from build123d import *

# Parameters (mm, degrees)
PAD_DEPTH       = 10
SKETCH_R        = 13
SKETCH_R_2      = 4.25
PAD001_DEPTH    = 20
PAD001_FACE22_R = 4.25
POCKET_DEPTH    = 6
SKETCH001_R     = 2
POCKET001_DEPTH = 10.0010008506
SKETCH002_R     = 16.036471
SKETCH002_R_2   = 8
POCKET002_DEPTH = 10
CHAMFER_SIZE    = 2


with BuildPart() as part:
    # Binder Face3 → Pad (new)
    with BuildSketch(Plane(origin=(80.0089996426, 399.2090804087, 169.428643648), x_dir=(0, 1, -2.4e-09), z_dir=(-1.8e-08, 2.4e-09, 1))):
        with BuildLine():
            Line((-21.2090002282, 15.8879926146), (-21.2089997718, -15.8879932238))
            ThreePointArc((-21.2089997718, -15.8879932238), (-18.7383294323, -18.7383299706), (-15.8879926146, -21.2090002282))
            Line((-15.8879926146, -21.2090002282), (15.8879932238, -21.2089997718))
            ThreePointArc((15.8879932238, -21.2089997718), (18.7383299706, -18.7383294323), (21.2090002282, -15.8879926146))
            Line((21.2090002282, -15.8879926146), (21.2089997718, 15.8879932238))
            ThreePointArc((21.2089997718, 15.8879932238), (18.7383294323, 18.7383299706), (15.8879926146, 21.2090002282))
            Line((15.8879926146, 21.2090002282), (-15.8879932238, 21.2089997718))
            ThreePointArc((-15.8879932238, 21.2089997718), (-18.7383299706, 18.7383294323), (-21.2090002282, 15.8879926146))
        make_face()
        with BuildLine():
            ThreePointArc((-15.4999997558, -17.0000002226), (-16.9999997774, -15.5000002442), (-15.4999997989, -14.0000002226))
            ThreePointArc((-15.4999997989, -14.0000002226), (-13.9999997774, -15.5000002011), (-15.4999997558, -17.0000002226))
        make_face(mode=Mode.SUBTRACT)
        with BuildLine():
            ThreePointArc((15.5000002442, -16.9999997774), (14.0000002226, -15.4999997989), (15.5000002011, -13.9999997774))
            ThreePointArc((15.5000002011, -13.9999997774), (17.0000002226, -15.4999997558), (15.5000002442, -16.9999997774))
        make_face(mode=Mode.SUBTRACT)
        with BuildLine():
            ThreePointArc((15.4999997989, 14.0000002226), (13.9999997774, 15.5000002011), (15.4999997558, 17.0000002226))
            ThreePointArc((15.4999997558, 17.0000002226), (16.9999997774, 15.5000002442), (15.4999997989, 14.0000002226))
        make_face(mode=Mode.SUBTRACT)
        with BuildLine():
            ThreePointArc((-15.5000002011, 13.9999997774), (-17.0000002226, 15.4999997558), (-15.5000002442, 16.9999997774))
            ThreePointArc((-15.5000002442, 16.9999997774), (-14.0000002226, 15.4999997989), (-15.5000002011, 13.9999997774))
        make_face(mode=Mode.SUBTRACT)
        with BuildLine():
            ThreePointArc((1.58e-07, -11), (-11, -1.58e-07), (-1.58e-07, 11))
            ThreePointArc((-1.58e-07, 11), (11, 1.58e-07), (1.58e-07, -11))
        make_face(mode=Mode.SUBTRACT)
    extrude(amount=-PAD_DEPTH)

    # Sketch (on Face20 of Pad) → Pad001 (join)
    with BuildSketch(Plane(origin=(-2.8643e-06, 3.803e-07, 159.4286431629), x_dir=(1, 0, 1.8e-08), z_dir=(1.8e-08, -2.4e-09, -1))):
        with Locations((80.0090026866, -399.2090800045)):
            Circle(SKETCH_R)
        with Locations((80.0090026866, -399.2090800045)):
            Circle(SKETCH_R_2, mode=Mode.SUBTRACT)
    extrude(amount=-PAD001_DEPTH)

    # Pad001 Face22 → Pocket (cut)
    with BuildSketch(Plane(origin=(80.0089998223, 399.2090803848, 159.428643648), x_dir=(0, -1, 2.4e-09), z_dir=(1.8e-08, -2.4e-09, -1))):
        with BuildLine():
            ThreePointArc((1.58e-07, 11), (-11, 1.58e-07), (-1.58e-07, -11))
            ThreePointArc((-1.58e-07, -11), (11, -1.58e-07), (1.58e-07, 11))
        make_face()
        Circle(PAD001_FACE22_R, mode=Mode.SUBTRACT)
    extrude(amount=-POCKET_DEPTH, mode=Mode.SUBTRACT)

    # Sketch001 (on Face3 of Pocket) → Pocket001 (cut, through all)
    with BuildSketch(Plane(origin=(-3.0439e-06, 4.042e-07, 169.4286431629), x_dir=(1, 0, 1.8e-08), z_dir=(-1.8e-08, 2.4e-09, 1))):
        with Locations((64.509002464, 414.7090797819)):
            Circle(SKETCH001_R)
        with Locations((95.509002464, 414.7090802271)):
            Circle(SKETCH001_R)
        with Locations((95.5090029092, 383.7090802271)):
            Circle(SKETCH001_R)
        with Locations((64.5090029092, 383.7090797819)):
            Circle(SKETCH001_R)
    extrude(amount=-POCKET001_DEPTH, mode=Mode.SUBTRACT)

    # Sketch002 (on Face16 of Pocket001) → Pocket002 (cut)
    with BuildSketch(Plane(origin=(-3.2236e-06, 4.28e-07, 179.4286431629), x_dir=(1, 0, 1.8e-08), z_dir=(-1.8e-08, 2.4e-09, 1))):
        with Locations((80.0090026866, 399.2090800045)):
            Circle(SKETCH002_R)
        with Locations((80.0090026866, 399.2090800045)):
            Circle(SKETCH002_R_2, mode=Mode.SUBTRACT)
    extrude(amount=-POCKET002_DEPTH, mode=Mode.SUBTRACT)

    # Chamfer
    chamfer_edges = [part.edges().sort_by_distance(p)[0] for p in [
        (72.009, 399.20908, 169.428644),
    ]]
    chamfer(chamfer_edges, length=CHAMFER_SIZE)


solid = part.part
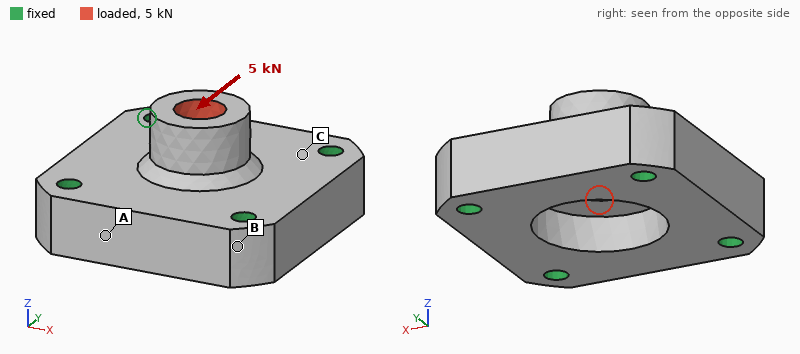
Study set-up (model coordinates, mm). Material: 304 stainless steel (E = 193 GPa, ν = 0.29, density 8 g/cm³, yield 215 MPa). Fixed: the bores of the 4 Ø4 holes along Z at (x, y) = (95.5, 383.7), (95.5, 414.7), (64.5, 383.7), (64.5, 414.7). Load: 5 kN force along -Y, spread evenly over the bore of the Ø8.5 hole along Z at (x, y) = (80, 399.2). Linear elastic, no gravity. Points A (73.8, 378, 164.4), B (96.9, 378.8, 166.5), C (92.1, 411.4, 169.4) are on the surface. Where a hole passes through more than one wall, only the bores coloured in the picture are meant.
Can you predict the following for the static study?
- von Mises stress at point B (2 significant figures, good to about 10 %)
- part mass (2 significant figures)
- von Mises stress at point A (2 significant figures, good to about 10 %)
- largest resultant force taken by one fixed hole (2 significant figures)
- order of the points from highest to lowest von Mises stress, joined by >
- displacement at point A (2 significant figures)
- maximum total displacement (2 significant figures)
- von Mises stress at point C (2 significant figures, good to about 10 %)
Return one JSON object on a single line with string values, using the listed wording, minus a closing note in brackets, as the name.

{"von Mises stress at point B": "5.9 MPa", "part mass": "130 g", "von Mises stress at point A": "10.0 MPa", "largest resultant force taken by one fixed hole": "1.5 kN", "order of the points from highest to lowest von Mises stress, joined by >": "C > A > B", "displacement at point A": "1.2 µm", "maximum total displacement": "7.6 µm", "von Mises stress at point C": "20 MPa"}
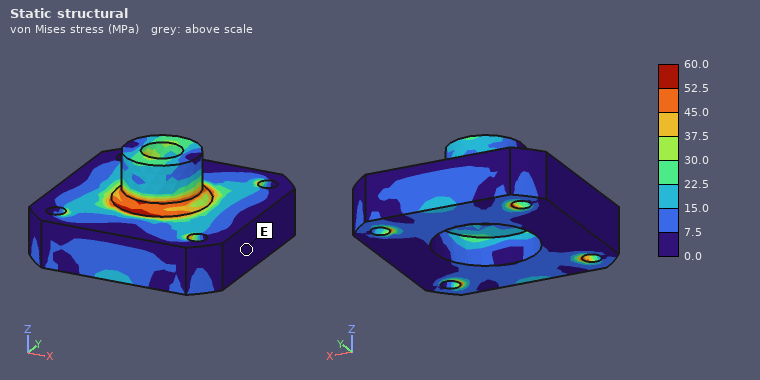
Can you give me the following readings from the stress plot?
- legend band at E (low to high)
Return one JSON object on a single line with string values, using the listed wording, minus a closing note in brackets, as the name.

{"legend band at E": "0.0 to 7.5 MPa"}
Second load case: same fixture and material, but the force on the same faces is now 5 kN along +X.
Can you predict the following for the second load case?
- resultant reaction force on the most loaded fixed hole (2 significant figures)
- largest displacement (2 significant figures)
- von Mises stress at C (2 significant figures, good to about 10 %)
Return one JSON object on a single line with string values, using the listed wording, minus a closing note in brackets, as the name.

{"resultant reaction force on the most loaded fixed hole": "1.5 kN", "largest displacement": "7.6 µm", "von Mises stress at C": "20 MPa"}
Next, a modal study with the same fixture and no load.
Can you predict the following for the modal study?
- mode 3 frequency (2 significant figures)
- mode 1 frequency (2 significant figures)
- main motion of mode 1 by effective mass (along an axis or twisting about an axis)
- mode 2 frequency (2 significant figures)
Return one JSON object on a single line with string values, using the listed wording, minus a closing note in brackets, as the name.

{"mode 3 frequency": "31 kHz", "mode 1 frequency": "26 kHz", "main motion of mode 1 by effective mass": "along Z", "mode 2 frequency": "31 kHz"}
